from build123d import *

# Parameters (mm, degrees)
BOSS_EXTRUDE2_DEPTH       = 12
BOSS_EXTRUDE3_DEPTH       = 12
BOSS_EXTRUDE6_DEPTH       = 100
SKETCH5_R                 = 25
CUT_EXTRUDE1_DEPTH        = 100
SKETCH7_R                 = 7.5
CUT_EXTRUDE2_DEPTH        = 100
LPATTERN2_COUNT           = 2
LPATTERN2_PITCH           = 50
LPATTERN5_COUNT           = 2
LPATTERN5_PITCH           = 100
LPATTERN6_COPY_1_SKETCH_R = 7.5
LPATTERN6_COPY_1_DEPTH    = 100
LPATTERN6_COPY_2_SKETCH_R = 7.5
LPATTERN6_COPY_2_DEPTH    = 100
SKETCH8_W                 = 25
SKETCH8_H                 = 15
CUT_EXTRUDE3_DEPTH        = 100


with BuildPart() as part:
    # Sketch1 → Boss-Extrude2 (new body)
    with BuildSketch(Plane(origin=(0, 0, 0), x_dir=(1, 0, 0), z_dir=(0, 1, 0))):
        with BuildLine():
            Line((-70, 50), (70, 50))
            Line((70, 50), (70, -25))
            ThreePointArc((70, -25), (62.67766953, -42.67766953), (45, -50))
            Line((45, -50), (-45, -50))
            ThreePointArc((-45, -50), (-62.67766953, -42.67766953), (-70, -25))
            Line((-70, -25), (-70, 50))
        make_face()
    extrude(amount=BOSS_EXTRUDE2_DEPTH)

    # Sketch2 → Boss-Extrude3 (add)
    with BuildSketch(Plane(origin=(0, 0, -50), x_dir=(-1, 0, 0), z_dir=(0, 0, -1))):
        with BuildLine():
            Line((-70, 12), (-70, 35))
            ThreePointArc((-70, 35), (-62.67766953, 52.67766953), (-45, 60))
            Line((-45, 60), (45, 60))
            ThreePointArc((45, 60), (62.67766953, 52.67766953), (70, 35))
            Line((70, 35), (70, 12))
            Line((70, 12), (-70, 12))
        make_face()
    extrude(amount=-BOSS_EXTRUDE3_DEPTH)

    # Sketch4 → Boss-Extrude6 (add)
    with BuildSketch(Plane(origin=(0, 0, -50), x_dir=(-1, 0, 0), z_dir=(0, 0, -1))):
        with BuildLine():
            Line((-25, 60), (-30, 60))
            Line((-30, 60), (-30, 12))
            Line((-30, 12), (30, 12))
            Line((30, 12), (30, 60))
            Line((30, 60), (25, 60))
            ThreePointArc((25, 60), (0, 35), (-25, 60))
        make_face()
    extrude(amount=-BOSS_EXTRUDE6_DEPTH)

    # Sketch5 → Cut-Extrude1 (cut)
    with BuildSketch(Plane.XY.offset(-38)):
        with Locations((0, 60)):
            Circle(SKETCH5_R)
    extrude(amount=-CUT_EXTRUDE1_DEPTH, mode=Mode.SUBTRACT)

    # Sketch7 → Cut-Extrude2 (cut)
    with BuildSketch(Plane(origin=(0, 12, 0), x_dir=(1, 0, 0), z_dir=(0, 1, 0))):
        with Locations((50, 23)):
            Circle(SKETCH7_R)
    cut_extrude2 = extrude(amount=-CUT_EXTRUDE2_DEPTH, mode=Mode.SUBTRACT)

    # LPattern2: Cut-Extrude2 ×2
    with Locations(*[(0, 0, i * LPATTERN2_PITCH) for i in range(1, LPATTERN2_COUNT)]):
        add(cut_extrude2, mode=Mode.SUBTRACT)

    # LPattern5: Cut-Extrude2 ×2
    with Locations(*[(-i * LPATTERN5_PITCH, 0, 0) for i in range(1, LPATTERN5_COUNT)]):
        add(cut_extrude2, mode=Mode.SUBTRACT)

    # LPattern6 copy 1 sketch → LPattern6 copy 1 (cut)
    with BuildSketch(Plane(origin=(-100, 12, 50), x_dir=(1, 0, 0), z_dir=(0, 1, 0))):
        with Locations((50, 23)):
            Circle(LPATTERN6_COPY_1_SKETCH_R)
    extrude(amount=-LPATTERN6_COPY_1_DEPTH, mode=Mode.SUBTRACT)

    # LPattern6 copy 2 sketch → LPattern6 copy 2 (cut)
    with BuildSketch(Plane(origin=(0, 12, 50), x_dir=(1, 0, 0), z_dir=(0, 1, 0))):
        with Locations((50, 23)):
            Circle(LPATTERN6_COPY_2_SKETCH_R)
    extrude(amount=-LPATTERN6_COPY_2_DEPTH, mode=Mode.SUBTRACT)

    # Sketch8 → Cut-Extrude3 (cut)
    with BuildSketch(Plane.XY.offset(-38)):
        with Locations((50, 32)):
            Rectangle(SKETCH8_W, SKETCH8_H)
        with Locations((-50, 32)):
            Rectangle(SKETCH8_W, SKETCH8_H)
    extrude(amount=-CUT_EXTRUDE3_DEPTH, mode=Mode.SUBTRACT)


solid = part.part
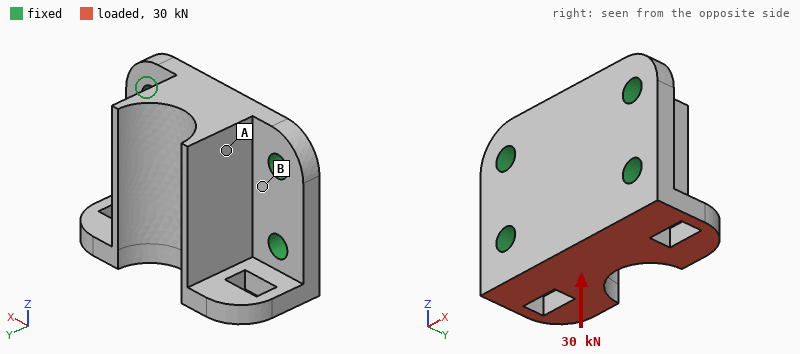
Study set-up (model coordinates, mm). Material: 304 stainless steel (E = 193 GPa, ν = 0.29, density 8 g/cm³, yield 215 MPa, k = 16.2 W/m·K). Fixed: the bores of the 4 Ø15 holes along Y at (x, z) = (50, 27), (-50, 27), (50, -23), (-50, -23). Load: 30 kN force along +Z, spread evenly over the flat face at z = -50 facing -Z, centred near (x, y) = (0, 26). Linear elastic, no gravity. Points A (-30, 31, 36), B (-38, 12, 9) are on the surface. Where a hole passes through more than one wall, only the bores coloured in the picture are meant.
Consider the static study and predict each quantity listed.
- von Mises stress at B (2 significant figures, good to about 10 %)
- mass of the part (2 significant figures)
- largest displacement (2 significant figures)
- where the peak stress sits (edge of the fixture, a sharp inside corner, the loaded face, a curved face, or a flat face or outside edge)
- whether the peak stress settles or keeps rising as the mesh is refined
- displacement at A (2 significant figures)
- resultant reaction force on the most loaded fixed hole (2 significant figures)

30 MPa
3.0 kg
62 µm
edge of the fixture
keeps rising
13 µm
11 kN
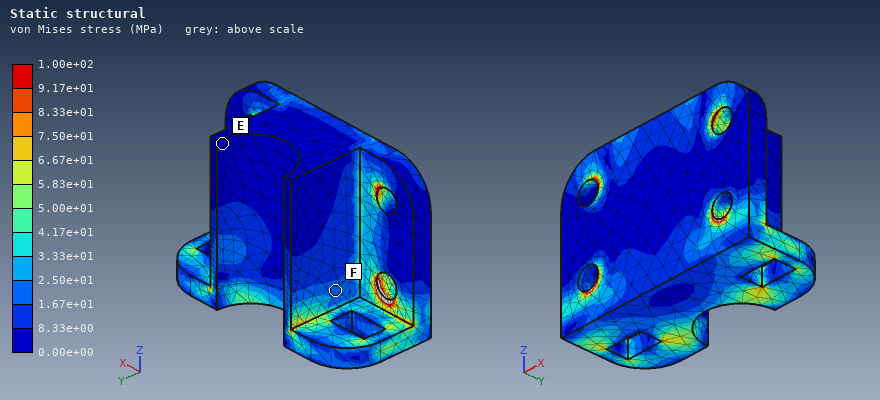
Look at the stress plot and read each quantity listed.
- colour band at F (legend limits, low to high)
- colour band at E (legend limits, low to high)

1.67e+01 to 2.50e+01 MPa
0.00e+00 to 8.33e+00 MPa
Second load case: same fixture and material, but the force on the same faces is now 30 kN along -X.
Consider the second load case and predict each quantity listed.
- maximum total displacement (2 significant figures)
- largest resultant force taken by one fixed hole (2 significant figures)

27 µm
15 kN
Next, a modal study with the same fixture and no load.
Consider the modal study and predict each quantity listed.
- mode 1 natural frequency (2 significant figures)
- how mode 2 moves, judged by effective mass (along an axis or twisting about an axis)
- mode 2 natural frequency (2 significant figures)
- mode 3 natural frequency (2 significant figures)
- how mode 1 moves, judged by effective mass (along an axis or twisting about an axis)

4000 Hz
along Y
5700 Hz
6200 Hz
along Z
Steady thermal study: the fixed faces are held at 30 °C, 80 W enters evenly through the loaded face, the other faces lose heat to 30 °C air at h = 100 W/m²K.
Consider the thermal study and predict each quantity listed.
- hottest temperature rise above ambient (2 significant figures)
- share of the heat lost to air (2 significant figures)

42 K
66 %
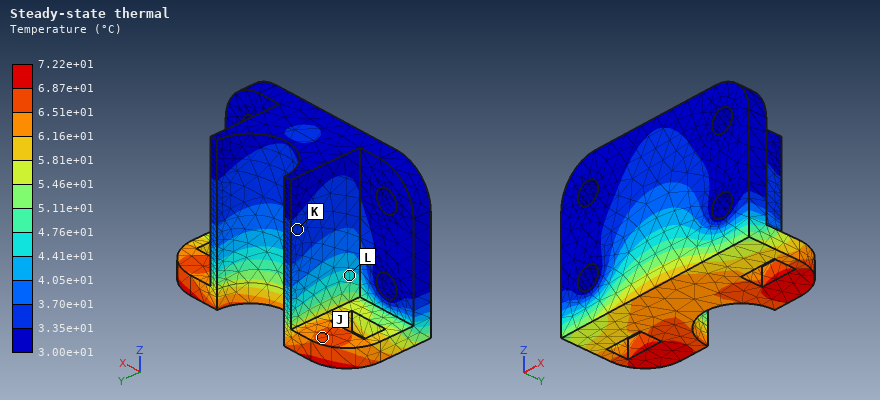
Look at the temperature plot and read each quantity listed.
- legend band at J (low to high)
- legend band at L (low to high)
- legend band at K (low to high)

6.51e+01 to 6.87e+01 °C
4.41e+01 to 4.76e+01 °C
3.35e+01 to 3.70e+01 °C
